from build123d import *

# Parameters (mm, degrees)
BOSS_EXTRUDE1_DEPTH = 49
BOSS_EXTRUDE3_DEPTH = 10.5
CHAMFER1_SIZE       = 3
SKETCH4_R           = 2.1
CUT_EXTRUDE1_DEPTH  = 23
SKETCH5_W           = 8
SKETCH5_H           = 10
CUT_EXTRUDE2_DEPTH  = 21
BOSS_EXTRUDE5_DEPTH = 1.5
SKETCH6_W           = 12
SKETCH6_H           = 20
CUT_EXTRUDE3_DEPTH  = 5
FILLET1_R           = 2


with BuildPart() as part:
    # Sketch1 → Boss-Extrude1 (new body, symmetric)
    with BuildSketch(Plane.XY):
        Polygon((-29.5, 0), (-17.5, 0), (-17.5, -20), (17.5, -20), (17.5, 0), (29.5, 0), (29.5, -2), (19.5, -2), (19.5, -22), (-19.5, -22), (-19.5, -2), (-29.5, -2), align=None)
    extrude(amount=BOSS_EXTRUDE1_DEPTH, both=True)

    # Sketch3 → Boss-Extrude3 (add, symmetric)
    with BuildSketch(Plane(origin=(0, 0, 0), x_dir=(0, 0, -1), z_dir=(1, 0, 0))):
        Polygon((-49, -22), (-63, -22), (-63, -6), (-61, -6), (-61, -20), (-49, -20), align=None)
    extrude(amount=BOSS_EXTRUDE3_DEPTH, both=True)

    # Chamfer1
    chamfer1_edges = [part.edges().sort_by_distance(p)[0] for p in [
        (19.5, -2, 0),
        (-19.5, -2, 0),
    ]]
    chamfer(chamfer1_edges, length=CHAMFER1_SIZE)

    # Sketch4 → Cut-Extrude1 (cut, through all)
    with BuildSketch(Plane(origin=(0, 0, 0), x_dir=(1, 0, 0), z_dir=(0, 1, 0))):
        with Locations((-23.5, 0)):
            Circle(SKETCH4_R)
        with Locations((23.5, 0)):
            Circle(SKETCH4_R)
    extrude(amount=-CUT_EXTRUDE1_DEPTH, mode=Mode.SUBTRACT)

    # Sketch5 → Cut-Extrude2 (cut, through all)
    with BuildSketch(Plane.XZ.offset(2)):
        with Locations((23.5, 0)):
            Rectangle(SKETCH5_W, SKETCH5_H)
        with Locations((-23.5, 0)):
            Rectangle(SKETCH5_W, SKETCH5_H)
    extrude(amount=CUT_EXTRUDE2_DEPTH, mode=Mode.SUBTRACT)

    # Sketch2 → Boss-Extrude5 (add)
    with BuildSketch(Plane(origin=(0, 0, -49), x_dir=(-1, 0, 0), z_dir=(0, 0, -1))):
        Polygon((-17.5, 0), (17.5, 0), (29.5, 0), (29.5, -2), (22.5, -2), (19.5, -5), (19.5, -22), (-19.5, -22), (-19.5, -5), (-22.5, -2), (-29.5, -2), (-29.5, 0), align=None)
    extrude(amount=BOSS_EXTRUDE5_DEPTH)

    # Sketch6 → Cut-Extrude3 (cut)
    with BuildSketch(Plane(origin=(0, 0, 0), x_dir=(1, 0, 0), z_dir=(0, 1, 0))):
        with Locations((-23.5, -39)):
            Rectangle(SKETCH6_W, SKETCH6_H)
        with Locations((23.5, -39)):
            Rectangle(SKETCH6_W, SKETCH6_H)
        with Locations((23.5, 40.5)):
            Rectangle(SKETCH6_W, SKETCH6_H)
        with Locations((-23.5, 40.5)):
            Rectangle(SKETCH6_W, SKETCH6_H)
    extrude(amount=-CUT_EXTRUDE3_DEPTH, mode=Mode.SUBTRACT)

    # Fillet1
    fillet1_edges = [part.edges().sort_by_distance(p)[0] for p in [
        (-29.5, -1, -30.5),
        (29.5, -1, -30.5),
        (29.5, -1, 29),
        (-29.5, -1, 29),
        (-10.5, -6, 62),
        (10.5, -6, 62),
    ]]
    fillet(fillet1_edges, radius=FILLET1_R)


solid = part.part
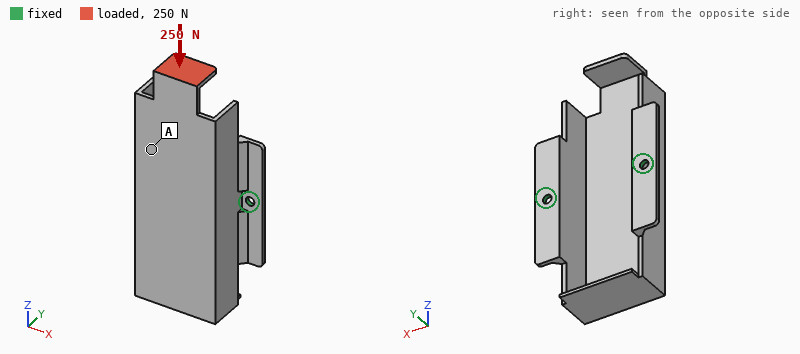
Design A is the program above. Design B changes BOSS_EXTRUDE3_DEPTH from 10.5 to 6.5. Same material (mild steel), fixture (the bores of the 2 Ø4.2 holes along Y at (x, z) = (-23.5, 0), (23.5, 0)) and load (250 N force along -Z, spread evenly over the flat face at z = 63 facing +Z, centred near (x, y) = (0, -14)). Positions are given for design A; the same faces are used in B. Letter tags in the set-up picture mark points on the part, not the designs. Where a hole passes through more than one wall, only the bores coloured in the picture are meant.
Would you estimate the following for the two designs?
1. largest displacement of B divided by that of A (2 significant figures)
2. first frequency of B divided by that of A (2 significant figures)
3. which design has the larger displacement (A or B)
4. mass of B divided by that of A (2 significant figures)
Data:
1.6
1.0
B
0.98
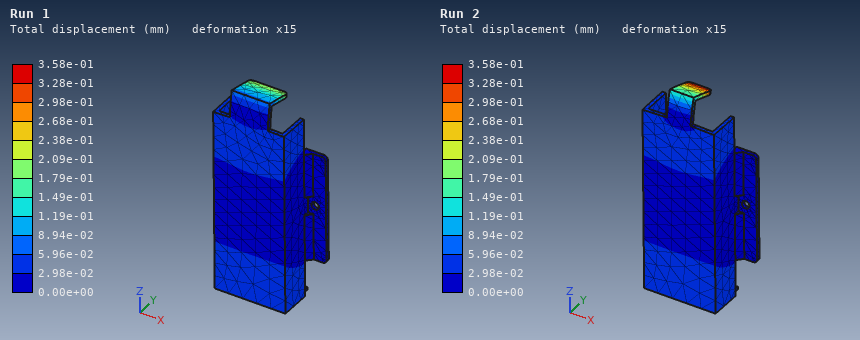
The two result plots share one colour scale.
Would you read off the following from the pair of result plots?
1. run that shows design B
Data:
Run 2
